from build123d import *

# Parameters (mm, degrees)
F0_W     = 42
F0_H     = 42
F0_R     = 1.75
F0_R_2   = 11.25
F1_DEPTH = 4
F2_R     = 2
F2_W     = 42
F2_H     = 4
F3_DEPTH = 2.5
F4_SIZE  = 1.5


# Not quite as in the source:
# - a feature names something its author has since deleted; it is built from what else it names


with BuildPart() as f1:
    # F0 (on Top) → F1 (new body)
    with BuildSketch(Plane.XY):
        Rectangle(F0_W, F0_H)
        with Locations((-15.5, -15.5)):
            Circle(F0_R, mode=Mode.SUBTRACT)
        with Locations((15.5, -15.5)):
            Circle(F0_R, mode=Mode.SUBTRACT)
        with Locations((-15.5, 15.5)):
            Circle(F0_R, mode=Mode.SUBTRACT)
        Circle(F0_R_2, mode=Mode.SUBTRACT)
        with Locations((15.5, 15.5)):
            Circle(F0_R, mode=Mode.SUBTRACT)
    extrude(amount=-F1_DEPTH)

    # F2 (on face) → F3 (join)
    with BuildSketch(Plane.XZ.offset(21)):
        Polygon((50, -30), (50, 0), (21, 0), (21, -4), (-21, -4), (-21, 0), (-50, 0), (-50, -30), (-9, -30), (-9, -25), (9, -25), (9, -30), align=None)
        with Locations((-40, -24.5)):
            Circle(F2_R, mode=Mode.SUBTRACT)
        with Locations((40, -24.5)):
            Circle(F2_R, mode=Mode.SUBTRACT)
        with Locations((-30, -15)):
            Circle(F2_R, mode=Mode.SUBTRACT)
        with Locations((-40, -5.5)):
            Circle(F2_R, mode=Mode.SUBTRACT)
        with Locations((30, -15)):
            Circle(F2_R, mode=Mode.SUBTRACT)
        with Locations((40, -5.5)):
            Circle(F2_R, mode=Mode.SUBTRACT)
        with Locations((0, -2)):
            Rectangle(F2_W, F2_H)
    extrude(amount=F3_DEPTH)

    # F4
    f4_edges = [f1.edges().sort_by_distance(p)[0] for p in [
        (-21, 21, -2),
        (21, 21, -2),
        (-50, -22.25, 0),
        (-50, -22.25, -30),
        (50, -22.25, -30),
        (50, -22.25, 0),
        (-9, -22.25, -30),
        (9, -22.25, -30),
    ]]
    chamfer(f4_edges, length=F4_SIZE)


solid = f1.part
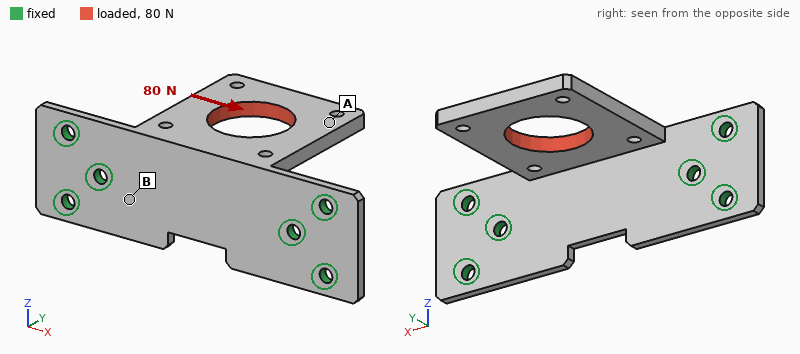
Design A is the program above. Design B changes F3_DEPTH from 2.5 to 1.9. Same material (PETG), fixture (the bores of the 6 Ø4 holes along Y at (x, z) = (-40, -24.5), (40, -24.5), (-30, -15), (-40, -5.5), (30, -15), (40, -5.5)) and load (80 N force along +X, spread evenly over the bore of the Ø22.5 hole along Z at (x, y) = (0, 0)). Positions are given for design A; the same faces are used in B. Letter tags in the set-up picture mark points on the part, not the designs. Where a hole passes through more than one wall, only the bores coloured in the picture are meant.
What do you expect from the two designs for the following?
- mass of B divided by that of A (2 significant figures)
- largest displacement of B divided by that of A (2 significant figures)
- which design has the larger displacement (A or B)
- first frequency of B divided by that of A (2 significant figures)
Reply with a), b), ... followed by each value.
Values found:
a) 0.86
b) 1.7
c) B
d) 0.75
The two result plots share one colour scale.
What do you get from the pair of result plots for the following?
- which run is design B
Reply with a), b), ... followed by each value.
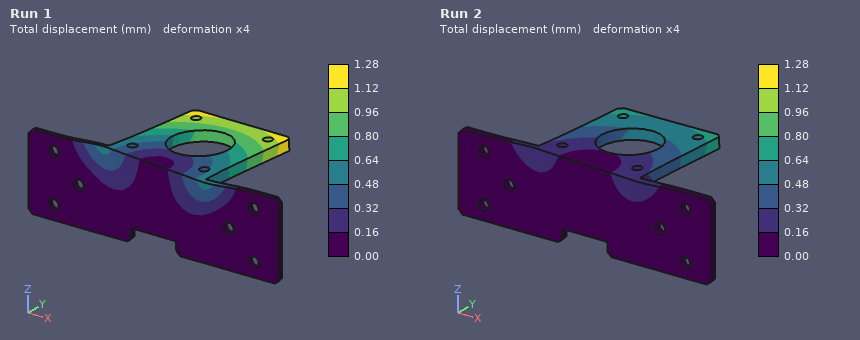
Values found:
a) Run 1
